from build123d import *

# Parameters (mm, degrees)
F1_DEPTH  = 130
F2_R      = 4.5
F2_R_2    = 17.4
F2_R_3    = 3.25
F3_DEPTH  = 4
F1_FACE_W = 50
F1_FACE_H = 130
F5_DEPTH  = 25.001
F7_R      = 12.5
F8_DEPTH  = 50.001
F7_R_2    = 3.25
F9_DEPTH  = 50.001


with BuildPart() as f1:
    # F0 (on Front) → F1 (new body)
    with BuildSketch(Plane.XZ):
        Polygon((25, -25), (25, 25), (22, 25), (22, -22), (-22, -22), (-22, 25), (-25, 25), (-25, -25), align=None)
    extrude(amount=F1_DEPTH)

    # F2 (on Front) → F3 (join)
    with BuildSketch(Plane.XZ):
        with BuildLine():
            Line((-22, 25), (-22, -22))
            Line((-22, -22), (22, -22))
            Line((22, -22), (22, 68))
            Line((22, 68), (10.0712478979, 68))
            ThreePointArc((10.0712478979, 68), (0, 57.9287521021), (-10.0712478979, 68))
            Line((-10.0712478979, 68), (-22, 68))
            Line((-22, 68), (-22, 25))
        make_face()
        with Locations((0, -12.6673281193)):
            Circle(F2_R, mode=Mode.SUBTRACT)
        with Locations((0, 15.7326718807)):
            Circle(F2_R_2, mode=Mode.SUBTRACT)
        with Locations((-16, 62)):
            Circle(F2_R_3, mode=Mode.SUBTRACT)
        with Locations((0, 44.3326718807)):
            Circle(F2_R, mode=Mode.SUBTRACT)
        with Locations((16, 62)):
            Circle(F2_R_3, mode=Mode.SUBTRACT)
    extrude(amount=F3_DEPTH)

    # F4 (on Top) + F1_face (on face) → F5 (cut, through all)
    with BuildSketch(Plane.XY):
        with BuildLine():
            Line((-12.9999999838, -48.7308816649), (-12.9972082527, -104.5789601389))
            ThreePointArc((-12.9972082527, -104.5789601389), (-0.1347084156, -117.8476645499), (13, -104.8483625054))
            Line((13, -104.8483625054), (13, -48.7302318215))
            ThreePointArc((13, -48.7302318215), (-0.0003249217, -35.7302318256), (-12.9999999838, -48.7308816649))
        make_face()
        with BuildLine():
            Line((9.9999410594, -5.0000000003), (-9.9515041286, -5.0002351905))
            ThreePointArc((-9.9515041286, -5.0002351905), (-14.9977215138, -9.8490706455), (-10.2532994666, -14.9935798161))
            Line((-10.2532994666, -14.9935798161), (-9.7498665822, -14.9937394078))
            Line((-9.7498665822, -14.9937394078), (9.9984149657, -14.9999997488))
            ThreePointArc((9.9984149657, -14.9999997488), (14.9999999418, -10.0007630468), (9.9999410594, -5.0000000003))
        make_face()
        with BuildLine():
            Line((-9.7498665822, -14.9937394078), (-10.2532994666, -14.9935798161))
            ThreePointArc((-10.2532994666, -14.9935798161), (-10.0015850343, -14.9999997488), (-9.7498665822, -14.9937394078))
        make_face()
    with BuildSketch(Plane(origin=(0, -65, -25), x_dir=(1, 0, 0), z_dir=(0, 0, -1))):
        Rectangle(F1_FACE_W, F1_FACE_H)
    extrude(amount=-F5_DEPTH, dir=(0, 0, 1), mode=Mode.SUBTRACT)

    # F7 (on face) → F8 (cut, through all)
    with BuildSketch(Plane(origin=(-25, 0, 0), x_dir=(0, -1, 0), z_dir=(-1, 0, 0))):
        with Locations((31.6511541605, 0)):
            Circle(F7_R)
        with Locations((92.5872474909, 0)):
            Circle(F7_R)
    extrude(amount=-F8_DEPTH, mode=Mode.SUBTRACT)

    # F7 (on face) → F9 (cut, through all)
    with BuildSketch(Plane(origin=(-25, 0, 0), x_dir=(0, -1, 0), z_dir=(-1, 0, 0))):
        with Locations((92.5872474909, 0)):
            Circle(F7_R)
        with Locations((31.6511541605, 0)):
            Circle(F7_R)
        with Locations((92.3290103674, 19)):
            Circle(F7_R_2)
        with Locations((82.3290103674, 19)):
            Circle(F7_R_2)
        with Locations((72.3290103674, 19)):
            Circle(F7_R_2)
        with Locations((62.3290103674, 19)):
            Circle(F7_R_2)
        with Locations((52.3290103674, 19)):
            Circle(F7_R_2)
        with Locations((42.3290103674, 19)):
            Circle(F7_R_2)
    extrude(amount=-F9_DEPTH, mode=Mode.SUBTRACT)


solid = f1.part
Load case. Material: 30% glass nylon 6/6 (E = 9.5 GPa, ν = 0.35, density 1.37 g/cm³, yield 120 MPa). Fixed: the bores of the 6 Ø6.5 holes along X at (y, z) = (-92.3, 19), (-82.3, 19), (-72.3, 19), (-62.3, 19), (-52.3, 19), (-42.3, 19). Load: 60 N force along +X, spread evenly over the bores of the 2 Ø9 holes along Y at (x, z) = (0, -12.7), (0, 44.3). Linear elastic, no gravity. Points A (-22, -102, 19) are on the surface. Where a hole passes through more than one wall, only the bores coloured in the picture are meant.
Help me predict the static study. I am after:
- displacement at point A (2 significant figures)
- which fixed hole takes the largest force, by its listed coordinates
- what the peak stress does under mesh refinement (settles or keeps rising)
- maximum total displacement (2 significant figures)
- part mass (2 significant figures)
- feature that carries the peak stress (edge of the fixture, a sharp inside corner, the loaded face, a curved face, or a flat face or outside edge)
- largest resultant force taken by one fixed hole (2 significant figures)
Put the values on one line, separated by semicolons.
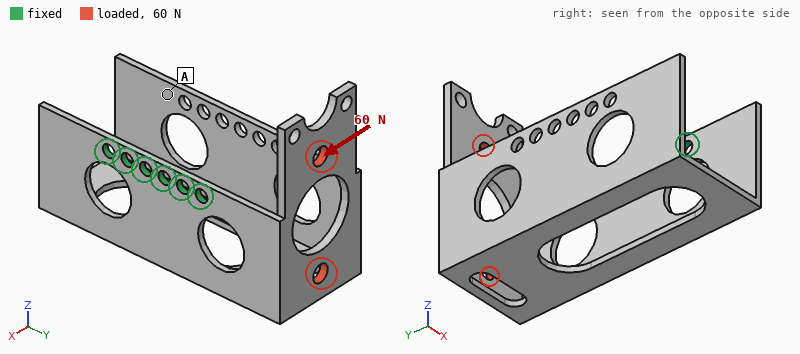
0.88 mm; (-42.3, 19); keeps rising; 1.5 mm; 72 g; edge of the fixture; 79 N
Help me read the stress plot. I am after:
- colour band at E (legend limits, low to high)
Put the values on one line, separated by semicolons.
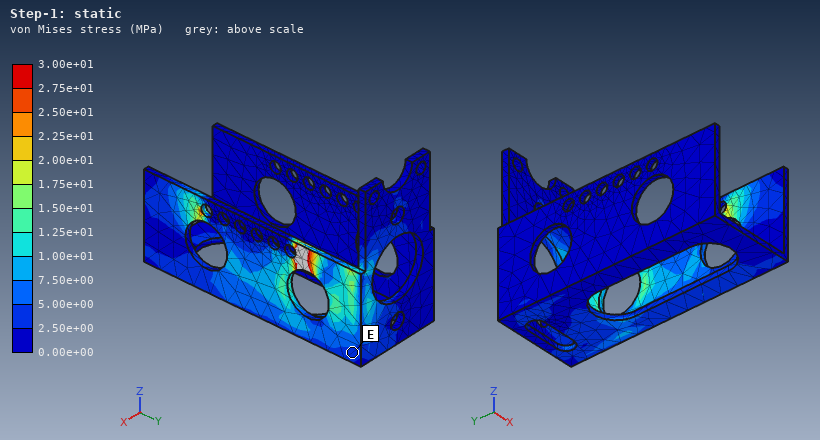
2.50e+00 to 5.00e+00 MPa
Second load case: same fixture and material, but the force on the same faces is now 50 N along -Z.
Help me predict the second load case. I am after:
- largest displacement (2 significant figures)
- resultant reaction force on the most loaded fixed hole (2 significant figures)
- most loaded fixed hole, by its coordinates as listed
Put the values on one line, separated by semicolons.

1.7 mm; 79 N; (-42.3, 19)
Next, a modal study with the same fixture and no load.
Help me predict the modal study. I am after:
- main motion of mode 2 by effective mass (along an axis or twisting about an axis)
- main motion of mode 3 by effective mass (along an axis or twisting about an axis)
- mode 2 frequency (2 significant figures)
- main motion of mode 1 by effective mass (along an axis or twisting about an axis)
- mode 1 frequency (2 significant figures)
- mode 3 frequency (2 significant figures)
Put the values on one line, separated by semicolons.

along Y; along X; 140 Hz; along Z; 110 Hz; 230 Hz
